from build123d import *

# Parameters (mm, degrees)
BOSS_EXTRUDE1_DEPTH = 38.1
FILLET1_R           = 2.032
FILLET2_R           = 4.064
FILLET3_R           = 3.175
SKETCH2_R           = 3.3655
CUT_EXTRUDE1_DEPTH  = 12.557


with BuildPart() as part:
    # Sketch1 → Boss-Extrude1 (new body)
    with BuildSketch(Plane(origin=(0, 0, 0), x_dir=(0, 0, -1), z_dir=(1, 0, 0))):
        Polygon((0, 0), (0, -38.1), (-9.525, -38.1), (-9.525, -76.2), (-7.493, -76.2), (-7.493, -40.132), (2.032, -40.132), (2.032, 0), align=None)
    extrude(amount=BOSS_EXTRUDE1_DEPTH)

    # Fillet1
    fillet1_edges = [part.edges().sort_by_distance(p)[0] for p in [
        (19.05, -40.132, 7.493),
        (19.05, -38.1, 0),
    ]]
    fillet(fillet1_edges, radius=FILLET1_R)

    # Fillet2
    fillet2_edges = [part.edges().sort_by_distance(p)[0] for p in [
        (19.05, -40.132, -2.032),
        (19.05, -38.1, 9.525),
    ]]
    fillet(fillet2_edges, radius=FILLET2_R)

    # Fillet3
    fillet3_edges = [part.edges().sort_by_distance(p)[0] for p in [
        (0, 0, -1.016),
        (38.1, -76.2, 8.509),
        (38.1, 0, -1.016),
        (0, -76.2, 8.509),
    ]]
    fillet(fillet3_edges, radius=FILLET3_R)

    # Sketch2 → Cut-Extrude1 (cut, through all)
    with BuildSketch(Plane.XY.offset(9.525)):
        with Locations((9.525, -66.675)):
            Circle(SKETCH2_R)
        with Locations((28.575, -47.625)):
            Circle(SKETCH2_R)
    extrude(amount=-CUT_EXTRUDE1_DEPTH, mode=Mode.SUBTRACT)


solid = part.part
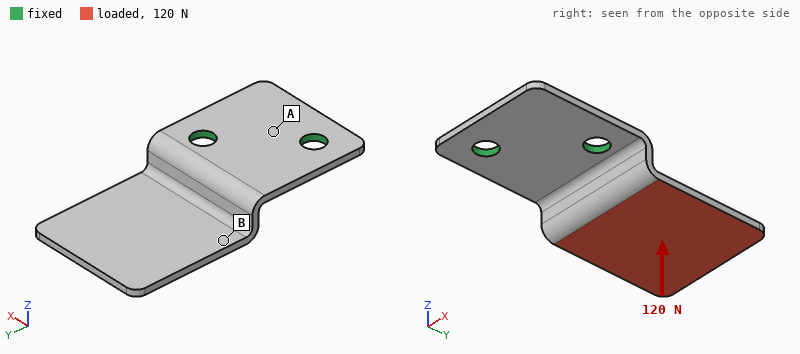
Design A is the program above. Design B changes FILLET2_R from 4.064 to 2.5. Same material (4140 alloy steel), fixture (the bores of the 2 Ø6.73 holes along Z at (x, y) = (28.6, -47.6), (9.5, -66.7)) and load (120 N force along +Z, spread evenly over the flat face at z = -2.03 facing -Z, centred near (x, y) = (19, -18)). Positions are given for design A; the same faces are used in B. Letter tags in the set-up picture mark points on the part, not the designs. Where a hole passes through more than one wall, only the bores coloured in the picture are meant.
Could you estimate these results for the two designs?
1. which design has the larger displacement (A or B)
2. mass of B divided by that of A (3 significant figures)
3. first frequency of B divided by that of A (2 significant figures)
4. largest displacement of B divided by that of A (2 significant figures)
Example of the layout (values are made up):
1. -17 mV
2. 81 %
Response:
1. A
2. 1.03
3. 1.0
4. 0.88
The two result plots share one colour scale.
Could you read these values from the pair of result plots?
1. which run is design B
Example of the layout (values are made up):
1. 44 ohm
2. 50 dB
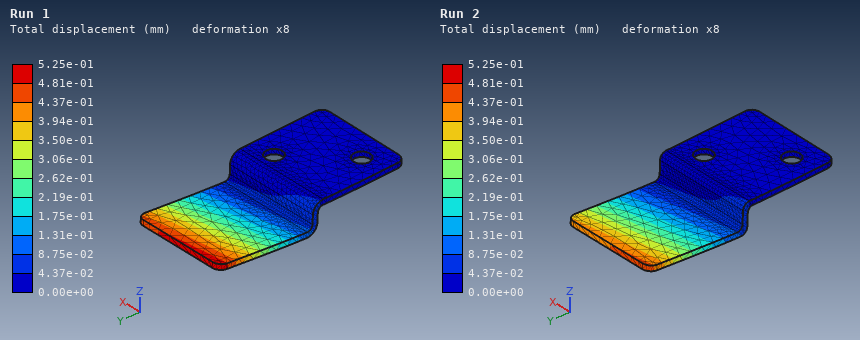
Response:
1. Run 2
